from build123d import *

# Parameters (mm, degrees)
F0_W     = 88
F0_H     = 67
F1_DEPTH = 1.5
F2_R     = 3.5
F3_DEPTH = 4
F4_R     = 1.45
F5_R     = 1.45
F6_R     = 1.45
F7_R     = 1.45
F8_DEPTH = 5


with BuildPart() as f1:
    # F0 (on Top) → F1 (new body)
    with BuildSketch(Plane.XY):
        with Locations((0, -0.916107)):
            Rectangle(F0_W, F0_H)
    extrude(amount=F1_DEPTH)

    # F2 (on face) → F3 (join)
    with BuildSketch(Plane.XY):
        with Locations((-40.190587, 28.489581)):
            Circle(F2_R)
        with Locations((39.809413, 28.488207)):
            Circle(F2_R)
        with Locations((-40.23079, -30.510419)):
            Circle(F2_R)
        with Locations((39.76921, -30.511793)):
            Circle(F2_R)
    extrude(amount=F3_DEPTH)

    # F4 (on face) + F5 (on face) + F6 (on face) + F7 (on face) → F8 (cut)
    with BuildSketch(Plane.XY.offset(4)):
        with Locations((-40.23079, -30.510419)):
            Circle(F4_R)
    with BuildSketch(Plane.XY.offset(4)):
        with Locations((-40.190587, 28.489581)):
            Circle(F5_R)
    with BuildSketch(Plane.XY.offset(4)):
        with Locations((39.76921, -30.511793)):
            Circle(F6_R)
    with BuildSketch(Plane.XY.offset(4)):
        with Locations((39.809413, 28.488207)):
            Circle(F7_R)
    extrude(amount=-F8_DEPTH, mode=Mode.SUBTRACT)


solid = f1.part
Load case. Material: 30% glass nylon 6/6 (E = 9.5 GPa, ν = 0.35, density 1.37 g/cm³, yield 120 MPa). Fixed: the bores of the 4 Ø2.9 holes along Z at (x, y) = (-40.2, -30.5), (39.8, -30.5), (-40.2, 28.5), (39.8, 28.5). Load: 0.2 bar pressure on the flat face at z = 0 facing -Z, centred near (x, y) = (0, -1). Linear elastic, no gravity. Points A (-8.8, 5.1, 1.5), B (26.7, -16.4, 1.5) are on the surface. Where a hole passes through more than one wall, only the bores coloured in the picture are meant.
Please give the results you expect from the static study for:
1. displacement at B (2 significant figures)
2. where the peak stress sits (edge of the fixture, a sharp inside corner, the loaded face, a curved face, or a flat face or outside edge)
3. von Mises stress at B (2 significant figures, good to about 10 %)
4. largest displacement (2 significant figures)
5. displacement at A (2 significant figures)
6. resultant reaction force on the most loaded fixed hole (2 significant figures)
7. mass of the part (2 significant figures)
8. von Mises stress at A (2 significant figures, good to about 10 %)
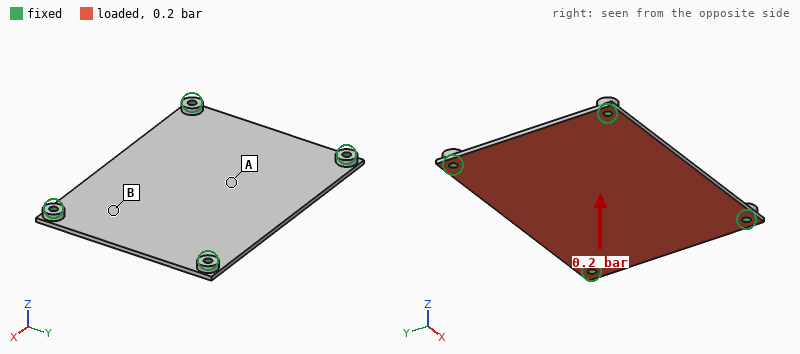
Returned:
0.50 mm
the loaded face
5.2 MPa
1.2 mm
1.1 mm
34 N
12 g
13 MPa
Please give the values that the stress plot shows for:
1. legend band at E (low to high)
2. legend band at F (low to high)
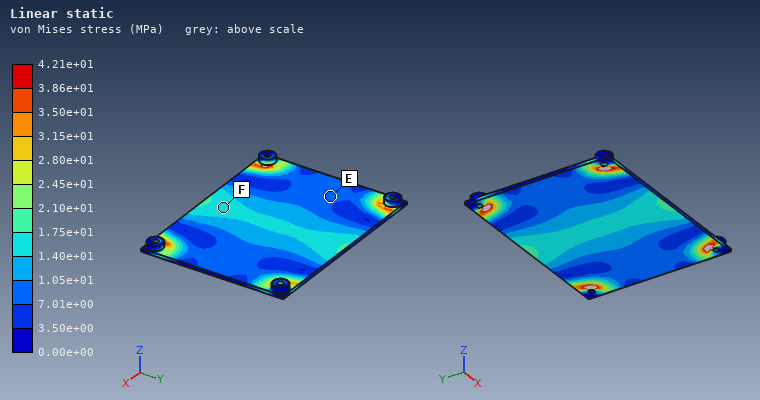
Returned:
7.01e+00 to 1.05e+01 MPa
1.40e+01 to 1.75e+01 MPa
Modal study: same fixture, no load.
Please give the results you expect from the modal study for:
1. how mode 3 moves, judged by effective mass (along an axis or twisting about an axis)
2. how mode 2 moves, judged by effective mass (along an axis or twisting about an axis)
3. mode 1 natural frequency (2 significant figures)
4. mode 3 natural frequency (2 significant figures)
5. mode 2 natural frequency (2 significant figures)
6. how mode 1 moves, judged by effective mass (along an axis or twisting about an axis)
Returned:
twisting about Y
twisting about X
540 Hz
1200 Hz
860 Hz
along Z
